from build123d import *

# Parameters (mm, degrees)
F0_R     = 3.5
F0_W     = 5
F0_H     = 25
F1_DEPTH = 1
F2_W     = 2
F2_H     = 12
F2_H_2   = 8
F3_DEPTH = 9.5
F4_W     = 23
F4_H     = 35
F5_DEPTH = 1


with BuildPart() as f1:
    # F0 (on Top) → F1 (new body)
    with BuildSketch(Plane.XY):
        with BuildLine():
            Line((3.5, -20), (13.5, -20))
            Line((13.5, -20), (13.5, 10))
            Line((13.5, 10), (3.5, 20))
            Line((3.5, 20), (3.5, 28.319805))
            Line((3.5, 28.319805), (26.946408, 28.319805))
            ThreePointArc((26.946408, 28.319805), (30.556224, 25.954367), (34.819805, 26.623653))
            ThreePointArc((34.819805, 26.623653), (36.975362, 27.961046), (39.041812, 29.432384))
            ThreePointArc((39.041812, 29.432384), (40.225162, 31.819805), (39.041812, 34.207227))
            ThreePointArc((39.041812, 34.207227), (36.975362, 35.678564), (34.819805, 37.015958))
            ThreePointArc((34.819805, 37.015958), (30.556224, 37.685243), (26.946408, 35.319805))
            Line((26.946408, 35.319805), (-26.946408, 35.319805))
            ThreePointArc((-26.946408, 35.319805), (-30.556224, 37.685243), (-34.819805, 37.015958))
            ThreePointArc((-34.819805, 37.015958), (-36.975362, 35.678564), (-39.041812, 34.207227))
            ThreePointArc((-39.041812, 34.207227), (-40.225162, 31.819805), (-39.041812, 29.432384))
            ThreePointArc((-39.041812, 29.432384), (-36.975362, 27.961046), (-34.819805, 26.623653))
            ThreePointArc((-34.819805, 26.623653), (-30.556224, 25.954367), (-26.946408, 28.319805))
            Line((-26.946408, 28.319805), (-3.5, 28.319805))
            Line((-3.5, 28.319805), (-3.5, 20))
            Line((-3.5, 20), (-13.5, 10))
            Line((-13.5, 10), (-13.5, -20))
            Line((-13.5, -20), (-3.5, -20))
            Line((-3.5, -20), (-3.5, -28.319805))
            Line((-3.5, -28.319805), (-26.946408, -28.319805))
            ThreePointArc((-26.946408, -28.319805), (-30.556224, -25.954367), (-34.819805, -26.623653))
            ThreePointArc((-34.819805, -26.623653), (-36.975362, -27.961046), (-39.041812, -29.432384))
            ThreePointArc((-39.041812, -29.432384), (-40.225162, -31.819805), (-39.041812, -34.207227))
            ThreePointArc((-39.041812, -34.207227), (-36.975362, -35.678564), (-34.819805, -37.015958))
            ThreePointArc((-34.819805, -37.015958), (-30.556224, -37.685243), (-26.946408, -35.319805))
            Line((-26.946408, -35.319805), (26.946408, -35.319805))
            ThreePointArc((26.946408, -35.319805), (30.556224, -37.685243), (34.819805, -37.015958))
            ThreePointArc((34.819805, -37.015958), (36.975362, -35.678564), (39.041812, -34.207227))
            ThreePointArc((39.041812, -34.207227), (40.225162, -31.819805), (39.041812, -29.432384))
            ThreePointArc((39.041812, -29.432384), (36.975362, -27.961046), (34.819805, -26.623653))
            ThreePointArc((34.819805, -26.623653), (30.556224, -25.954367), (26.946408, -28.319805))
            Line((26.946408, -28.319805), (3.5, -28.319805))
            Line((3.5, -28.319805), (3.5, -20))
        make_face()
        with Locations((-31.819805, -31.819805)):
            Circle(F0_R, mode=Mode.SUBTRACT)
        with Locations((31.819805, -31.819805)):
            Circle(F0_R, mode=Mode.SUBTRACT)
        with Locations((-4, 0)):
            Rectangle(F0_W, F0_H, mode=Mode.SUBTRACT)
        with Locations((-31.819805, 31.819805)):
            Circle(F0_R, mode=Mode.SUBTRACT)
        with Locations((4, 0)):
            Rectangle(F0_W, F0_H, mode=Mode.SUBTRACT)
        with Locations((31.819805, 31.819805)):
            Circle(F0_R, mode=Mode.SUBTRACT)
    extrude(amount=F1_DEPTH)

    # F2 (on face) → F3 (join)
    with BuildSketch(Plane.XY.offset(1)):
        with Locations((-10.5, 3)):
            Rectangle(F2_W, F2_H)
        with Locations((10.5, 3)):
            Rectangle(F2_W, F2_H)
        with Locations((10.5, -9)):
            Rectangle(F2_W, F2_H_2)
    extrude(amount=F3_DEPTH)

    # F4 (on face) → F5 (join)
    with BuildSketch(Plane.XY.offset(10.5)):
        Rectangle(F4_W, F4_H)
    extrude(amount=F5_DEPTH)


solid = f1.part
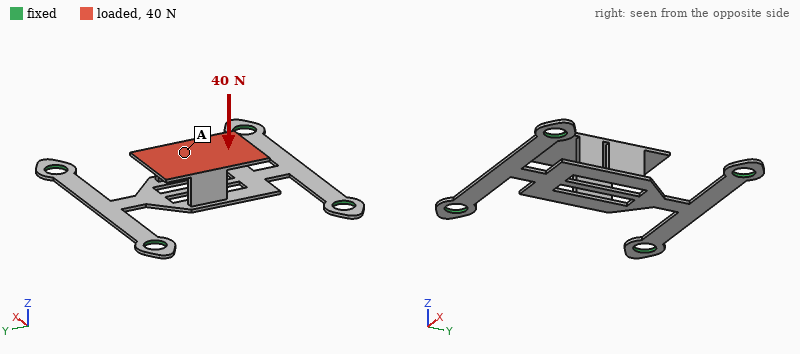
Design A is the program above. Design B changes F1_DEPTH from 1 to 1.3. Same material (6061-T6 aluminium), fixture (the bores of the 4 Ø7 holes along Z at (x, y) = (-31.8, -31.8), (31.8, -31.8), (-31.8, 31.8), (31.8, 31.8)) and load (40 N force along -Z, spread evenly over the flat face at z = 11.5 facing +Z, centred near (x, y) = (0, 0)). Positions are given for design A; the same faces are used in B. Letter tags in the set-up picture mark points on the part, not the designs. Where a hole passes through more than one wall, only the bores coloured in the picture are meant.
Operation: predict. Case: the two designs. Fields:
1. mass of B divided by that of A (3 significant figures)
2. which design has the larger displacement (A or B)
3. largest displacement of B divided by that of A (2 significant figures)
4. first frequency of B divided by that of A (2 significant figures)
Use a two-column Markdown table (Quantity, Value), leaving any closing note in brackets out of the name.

| Quantity | Value |
|---|---|
| mass of B divided by that of A | 1.17 |
| which design has the larger displacement | A |
| largest displacement of B divided by that of A | 0.47 |
| first frequency of B divided by that of A | 1.4 |
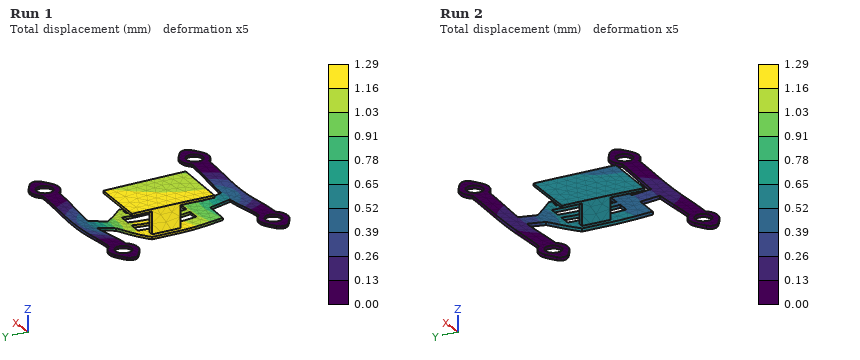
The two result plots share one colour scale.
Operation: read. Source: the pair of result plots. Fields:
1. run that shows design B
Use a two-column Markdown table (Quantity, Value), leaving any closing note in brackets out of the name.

| Quantity | Value |
|---|---|
| run that shows design B | Run 2 |
